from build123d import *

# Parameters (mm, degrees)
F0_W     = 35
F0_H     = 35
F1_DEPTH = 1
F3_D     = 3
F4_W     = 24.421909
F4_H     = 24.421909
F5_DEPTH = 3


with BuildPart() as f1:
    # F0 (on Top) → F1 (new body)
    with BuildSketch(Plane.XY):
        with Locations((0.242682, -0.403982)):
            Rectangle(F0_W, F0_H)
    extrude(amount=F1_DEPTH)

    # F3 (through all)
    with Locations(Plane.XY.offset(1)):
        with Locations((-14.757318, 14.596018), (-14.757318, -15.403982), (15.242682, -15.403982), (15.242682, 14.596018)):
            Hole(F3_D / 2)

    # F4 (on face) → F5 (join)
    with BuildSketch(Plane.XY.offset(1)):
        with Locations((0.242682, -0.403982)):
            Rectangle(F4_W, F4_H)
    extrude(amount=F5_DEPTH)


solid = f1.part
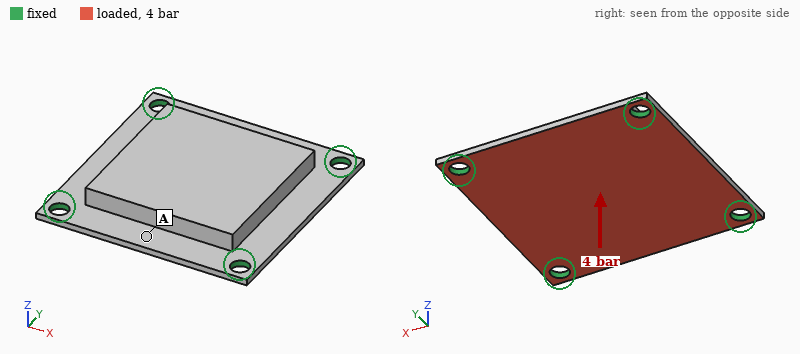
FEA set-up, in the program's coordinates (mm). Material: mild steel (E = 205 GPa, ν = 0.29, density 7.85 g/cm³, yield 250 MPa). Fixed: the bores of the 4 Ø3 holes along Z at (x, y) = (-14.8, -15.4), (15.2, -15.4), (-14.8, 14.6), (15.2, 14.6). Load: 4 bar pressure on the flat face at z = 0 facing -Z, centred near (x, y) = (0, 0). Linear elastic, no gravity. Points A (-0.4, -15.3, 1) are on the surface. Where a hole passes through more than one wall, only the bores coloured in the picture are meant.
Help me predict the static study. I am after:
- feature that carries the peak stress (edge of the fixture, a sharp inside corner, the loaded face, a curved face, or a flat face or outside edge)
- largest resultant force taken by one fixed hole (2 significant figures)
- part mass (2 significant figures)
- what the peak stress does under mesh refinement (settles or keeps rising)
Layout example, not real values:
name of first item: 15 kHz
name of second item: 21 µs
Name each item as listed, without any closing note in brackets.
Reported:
feature that carries the peak stress: edge of the fixture
largest resultant force taken by one fixed hole: 160 N
part mass: 23 g
what the peak stress does under mesh refinement: keeps rising
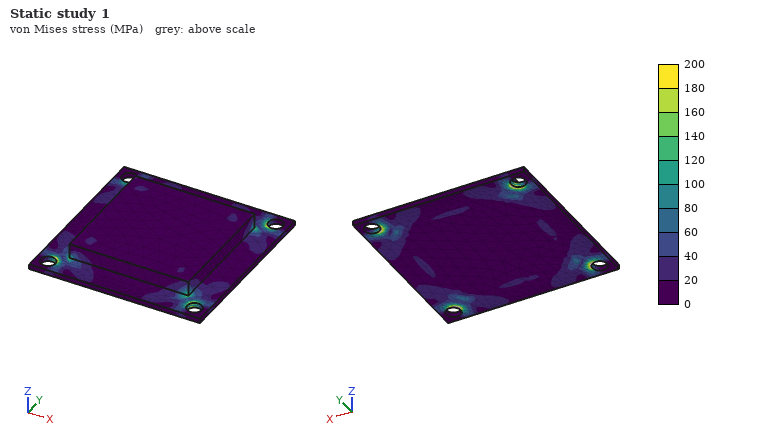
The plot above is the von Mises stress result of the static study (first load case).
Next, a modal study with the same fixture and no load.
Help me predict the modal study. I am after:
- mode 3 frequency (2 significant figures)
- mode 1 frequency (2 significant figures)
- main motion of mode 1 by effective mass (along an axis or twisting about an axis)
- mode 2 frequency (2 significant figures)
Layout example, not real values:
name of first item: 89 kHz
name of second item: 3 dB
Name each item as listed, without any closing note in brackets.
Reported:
mode 3 frequency: 12 kHz
mode 1 frequency: 7300 Hz
main motion of mode 1 by effective mass: along Z
mode 2 frequency: 12 kHz
